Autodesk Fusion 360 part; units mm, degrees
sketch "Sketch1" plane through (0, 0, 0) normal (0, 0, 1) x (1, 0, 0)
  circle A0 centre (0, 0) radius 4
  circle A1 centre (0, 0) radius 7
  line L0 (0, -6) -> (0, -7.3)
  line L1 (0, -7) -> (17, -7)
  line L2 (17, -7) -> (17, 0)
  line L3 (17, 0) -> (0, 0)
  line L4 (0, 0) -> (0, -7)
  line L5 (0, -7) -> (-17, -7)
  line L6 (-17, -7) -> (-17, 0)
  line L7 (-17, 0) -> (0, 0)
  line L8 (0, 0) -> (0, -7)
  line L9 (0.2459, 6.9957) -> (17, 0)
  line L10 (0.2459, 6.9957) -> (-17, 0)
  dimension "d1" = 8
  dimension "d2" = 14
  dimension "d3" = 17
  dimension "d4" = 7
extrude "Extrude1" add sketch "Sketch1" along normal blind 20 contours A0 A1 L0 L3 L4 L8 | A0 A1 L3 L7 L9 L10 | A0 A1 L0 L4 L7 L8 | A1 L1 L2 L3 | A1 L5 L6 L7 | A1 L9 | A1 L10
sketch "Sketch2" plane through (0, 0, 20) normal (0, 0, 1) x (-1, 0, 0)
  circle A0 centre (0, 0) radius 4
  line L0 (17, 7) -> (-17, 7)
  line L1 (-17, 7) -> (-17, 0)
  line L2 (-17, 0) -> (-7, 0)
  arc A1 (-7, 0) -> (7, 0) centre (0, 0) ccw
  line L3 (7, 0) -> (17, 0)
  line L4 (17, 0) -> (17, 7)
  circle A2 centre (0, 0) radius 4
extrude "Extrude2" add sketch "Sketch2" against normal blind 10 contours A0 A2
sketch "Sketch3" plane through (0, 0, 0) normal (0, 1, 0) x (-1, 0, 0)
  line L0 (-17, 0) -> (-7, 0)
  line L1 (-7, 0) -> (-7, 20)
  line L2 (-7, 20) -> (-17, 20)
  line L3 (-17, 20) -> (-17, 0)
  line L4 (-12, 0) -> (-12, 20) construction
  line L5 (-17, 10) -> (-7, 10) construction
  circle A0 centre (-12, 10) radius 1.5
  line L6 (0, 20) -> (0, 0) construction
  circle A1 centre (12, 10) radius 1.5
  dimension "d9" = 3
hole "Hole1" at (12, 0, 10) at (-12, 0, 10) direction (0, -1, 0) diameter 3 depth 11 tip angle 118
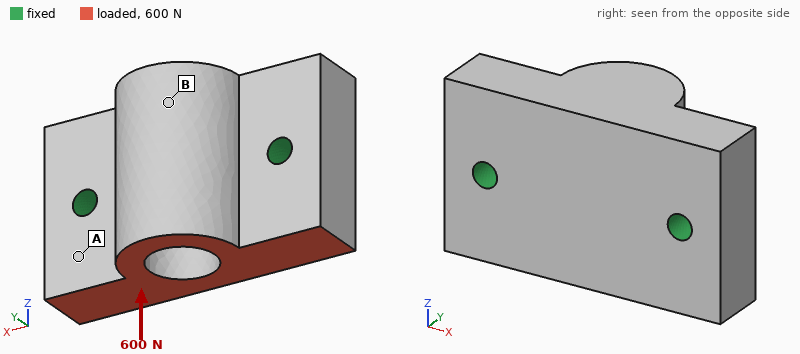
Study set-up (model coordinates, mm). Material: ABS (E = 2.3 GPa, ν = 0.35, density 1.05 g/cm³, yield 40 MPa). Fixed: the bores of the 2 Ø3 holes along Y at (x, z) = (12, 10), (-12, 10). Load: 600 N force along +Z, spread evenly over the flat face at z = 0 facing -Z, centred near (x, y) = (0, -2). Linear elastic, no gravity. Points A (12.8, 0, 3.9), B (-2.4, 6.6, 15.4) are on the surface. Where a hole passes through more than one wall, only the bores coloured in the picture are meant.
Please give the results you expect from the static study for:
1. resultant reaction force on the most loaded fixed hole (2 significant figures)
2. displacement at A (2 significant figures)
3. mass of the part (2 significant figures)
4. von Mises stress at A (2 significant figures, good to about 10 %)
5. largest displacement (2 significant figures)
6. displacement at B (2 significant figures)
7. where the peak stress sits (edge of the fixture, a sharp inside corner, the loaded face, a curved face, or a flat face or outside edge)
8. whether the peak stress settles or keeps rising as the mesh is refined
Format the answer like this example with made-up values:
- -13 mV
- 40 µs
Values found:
- 300 N
- 14 µm
- 6.0 g
- 3.6 MPa
- 61 µm
- 43 µm
- edge of the fixture
- keeps rising
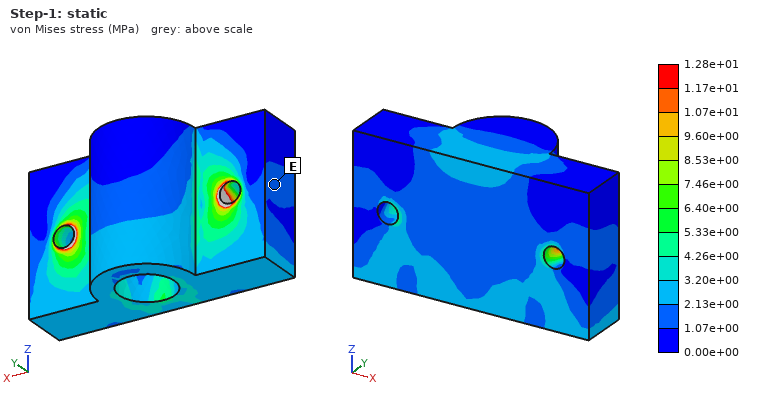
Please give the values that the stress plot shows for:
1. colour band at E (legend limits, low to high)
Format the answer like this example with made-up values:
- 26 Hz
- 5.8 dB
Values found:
- 1.07e+00 to 2.13e+00 MPa
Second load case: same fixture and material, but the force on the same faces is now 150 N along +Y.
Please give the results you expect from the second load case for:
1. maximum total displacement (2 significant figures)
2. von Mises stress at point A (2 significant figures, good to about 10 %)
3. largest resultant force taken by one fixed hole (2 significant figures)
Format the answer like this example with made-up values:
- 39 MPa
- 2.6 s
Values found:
- 63 µm
- 2.5 MPa
- 75 N
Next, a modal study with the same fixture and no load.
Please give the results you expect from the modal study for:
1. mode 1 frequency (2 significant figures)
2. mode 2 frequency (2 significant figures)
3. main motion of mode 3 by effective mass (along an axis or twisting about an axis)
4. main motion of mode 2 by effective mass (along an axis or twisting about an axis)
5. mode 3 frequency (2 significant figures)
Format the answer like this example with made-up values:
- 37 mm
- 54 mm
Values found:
- 6200 Hz
- 9200 Hz
- along Z
- along Y
- 12 kHz
